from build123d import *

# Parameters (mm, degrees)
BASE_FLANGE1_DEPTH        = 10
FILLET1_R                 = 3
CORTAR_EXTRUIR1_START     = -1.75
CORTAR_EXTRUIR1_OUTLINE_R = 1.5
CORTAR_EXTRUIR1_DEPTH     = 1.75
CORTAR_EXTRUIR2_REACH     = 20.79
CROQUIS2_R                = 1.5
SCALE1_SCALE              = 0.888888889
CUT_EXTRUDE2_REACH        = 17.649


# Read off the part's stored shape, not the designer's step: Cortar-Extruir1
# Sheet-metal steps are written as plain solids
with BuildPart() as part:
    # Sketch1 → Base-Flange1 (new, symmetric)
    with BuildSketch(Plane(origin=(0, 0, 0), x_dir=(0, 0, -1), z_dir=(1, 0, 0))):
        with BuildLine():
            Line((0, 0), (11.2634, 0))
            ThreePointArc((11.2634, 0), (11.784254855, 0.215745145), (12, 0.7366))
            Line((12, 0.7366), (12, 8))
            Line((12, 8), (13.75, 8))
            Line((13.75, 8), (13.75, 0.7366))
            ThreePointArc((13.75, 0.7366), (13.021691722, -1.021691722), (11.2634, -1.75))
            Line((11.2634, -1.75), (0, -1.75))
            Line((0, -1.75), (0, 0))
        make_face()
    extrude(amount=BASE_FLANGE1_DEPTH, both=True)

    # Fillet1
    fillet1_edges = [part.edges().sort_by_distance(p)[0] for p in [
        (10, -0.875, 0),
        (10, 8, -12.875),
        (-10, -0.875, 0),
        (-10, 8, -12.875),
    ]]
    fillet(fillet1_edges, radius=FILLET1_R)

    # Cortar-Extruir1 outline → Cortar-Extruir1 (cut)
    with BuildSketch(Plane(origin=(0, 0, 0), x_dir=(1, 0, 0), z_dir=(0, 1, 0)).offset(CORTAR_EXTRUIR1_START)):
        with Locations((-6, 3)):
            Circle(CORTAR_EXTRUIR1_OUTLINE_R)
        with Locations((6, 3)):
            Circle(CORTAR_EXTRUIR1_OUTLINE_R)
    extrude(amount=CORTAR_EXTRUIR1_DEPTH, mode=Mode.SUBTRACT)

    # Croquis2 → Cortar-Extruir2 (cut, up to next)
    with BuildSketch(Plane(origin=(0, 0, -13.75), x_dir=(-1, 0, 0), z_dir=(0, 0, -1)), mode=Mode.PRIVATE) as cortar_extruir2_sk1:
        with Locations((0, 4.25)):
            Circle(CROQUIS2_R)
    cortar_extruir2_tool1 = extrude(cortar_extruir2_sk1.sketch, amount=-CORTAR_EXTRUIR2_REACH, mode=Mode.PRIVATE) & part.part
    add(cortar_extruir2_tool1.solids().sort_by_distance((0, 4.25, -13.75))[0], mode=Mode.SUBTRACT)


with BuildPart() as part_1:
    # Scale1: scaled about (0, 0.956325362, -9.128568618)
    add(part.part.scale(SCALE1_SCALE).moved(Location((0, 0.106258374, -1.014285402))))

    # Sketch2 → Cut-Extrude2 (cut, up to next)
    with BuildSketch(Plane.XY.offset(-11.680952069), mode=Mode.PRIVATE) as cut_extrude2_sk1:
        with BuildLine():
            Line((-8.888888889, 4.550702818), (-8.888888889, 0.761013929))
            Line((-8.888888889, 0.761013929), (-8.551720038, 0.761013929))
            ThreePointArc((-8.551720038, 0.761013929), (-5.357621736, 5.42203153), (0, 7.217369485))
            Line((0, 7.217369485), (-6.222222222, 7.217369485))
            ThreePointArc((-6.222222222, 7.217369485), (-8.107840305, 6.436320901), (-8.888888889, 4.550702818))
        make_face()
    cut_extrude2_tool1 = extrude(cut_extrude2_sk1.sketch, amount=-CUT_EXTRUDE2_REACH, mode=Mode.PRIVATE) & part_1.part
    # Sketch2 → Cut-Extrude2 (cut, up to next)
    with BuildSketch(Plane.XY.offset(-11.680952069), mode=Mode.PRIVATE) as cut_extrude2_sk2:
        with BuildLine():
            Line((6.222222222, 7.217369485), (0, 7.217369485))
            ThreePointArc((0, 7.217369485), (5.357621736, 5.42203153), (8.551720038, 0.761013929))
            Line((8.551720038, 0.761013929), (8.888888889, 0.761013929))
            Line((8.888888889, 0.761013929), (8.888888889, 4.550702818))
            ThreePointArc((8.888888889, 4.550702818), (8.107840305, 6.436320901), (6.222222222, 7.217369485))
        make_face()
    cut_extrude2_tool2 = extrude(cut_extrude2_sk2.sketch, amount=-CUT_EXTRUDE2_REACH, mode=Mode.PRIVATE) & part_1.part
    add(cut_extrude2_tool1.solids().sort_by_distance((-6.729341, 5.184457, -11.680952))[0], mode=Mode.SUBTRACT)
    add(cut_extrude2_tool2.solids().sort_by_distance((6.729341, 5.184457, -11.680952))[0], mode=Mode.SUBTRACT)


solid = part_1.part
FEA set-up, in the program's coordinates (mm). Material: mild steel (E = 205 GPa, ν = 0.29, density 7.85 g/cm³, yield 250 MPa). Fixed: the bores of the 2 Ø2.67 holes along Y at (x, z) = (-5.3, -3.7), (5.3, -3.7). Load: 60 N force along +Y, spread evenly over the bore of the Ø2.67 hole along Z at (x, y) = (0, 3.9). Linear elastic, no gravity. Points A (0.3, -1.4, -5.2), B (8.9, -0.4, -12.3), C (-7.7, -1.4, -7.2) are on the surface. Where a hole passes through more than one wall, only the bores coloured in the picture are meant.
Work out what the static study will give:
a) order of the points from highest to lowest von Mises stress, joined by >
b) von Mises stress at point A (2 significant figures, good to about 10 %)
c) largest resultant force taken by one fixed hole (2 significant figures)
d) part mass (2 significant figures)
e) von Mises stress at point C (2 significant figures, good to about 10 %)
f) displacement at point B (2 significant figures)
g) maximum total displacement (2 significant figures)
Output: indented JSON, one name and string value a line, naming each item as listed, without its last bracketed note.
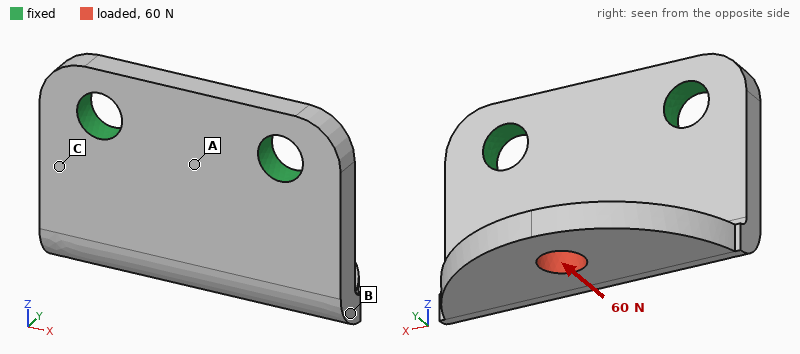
{
  "order of the points from highest to lowest von Mises stress, joined by >": "C > A > B",
  "von Mises stress at point A": "30 MPa",
  "largest resultant force taken by one fixed hole": "30 N",
  "part mass": "3.4 g",
  "von Mises stress at point C": "45 MPa",
  "displacement at point B": "9.2 µm",
  "maximum total displacement": "18 µm"
}
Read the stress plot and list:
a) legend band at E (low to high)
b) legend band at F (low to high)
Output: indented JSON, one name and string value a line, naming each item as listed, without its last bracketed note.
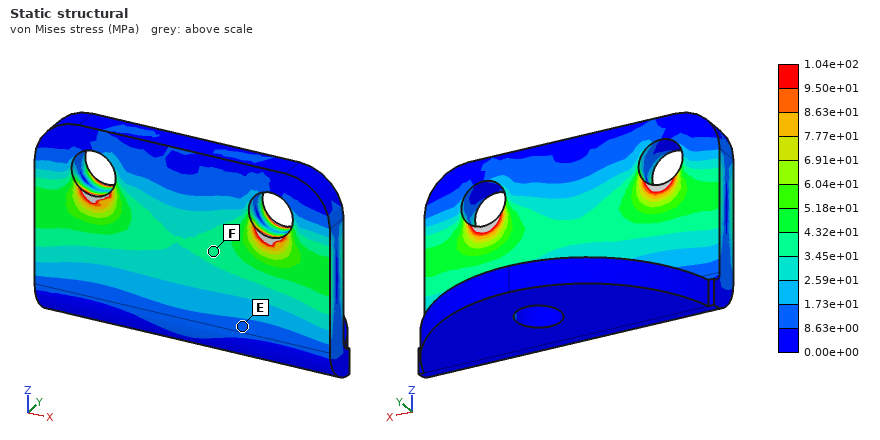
{
  "legend band at E": "8.63e+00 to 1.73e+01 MPa",
  "legend band at F": "3.45e+01 to 4.32e+01 MPa"
}
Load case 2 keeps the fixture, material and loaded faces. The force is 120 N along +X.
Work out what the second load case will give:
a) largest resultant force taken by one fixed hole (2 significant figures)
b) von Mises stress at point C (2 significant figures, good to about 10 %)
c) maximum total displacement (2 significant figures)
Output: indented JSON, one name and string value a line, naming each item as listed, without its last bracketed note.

{
  "largest resultant force taken by one fixed hole": "110 N",
  "von Mises stress at point C": "38 MPa",
  "maximum total displacement": "10.0 µm"
}
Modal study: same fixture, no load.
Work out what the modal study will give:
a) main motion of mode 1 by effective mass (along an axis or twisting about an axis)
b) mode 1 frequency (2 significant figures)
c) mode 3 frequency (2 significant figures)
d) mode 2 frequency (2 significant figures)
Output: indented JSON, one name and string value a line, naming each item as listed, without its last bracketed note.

{
  "main motion of mode 1 by effective mass": "along Y",
  "mode 1 frequency": "8400 Hz",
  "mode 3 frequency": "24 kHz",
  "mode 2 frequency": "15 kHz"
}
